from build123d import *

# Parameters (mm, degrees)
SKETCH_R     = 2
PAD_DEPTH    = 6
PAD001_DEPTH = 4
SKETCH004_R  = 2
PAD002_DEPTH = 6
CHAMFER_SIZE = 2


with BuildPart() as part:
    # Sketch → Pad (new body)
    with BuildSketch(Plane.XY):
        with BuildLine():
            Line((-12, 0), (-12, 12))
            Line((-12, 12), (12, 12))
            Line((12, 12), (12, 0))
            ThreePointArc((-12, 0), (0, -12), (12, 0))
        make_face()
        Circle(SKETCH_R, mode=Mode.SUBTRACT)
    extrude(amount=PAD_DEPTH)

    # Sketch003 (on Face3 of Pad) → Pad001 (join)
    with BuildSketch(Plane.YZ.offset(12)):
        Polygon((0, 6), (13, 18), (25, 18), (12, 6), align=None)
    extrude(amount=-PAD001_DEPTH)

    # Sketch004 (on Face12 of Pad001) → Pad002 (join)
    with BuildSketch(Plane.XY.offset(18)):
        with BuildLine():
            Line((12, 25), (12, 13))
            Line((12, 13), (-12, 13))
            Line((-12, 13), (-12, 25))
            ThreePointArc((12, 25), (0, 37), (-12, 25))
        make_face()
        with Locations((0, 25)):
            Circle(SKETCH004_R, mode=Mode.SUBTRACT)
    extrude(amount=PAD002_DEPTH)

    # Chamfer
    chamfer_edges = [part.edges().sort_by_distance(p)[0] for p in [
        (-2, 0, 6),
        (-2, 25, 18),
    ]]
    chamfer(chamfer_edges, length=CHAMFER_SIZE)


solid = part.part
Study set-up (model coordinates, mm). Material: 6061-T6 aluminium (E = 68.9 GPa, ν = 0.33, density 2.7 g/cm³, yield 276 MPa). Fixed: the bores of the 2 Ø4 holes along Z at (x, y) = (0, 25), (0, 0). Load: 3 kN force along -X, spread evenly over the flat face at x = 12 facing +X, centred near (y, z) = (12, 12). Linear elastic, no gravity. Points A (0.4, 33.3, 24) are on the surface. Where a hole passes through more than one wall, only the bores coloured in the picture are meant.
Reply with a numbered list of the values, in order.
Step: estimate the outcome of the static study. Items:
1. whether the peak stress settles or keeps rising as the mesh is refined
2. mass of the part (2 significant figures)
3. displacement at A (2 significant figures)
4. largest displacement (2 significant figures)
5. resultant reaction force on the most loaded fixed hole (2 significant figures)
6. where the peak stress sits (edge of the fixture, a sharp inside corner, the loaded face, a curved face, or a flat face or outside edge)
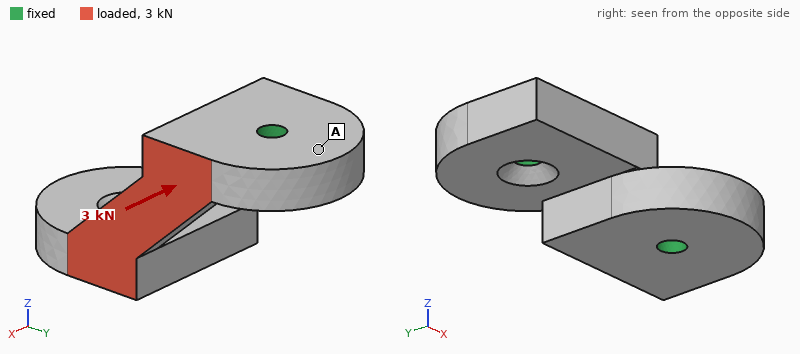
1. keeps rising
2. 18 g
3. 3.9 µm
4. 24 µm
5. 1.7 kN
6. edge of the fixture
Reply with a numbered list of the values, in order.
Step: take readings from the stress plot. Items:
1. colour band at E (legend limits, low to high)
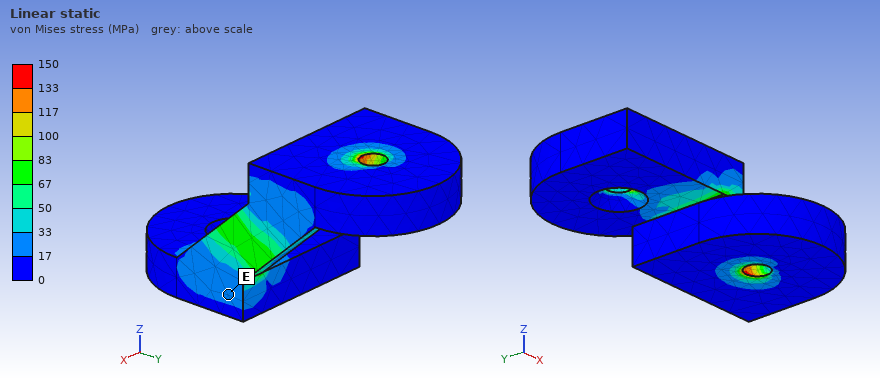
1. 17 to 33 MPa
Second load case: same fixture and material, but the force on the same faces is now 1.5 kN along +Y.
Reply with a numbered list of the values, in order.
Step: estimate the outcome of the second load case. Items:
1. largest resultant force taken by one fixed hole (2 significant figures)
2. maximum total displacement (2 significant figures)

1. 760 N
2. 32 µm
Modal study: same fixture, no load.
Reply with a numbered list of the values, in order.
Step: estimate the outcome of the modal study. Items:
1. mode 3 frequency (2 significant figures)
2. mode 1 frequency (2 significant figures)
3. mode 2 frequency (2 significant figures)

1. 17 kHz
2. 14 kHz
3. 17 kHz
